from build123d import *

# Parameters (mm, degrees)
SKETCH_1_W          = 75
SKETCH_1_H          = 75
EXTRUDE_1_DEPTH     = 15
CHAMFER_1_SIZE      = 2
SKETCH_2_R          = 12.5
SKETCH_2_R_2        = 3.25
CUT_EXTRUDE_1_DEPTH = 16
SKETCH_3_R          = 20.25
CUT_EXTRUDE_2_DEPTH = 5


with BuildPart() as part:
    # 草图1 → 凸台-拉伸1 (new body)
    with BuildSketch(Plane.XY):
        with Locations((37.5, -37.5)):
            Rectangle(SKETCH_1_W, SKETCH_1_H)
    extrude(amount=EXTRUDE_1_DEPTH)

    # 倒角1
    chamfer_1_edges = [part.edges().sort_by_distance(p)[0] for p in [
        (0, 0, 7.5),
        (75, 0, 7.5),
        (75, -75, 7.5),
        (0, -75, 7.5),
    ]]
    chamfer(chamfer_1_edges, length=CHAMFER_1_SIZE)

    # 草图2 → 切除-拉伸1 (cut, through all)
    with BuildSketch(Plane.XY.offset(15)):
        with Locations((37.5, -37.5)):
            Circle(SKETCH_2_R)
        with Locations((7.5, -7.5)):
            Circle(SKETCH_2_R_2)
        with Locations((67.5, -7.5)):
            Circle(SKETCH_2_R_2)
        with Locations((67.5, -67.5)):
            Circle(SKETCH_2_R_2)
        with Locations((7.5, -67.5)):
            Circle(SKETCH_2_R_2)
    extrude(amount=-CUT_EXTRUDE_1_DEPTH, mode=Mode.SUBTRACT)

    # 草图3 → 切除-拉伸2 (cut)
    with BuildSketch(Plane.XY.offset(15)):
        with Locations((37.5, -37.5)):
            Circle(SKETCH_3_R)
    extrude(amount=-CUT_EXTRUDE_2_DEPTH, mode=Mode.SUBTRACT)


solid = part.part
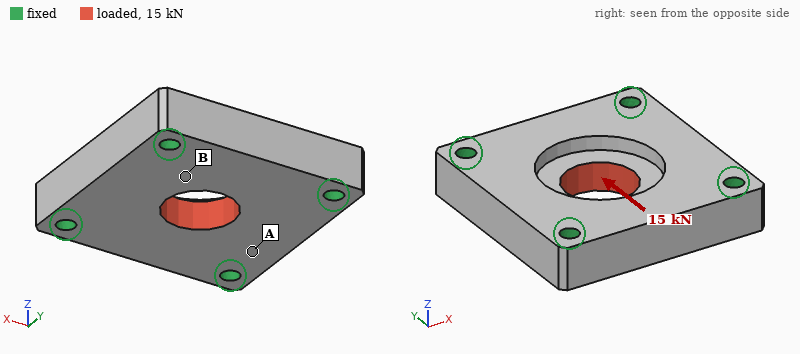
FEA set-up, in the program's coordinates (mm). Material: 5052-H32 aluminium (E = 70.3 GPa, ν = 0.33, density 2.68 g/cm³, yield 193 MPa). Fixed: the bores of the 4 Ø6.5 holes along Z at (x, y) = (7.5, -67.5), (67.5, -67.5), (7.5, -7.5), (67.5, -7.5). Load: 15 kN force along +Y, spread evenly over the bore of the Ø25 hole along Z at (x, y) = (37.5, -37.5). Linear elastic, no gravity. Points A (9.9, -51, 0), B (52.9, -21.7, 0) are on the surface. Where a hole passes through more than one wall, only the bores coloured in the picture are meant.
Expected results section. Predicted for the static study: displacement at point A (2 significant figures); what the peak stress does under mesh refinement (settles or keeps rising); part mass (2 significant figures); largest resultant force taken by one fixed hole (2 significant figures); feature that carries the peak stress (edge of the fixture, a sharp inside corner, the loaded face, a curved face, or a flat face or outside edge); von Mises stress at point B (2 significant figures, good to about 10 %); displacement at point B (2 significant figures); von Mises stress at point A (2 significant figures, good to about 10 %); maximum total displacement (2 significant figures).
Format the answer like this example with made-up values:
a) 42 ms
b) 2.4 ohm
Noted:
a) 2.6 µm
b) keeps rising
c) 190 g
d) 4.2 kN
e) edge of the fixture
f) 18 MPa
g) 6.2 µm
h) 10 MPa
i) 12 µm
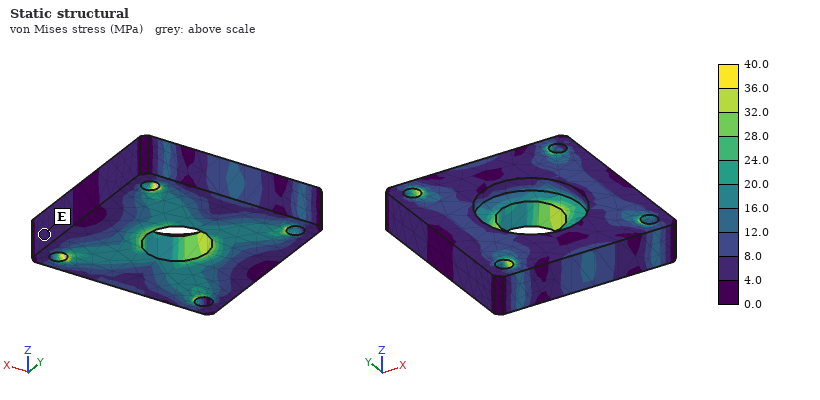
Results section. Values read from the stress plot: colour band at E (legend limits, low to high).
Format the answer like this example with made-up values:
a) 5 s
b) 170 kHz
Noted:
a) 4.0 to 8.0 MPa
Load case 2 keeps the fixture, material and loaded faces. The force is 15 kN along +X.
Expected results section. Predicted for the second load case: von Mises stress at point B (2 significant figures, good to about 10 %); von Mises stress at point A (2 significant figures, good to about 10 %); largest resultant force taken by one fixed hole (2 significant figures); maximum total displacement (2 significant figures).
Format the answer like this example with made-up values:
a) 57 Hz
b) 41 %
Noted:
a) 18 MPa
b) 15 MPa
c) 4.2 kN
d) 12 µm
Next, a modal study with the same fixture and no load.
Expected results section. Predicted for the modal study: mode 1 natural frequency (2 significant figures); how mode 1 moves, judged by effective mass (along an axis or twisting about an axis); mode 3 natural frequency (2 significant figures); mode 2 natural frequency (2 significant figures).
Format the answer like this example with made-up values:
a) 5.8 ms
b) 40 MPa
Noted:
a) 13 kHz
b) along Z
c) 17 kHz
d) 17 kHz
